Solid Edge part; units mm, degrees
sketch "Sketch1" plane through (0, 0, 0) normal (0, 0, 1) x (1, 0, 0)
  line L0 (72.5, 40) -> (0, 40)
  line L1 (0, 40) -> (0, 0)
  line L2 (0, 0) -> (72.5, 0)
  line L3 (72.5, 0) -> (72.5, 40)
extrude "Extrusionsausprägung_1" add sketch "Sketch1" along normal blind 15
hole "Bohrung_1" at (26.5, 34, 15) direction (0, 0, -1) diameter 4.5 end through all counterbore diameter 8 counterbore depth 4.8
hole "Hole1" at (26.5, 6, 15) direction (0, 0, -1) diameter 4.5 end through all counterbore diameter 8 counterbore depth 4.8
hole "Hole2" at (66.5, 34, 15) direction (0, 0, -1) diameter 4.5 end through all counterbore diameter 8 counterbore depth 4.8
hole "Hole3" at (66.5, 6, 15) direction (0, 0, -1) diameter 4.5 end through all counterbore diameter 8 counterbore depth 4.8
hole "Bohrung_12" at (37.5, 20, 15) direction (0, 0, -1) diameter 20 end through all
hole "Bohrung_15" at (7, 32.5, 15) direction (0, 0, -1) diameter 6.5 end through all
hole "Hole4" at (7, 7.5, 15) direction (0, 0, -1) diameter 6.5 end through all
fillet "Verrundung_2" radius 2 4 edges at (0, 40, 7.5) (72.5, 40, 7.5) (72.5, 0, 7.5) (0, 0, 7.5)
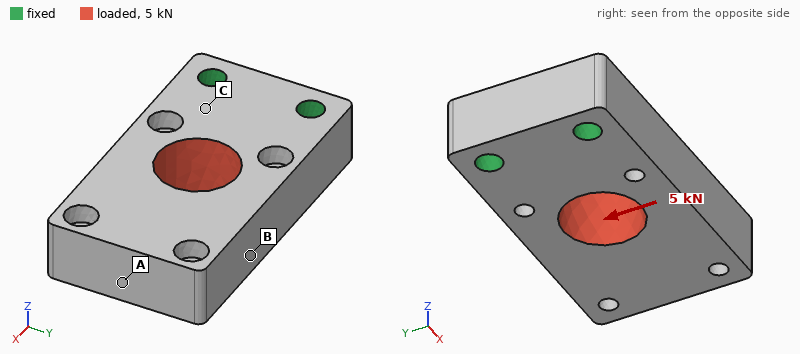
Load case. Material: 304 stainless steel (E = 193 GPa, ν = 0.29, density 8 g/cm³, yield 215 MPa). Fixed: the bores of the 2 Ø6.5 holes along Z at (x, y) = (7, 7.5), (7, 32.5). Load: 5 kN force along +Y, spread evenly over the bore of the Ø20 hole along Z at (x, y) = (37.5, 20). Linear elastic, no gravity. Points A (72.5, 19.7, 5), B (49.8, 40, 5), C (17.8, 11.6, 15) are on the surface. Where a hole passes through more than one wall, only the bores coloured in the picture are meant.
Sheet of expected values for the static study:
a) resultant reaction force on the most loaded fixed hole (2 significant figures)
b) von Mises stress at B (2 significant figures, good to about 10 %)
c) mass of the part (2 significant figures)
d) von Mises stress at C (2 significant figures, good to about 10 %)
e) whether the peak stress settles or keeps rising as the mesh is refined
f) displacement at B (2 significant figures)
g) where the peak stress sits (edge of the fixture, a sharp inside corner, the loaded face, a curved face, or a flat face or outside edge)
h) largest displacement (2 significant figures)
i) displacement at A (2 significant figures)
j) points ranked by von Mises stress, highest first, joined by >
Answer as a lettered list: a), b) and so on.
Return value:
a) 5.7 kN
b) 12 MPa
c) 290 g
d) 21 MPa
e) keeps rising
f) 16 µm
g) edge of the fixture
h) 20 µm
i) 20 µm
j) C > B > A
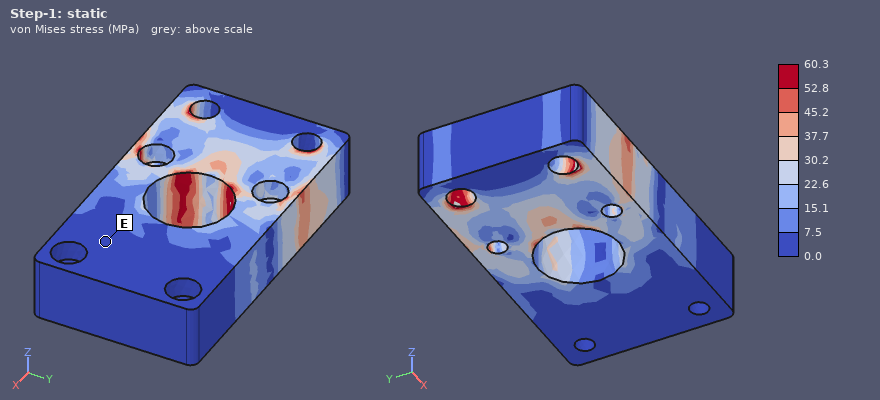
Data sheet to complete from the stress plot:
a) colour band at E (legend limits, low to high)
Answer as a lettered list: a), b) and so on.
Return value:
a) 0.0 to 7.5 MPa
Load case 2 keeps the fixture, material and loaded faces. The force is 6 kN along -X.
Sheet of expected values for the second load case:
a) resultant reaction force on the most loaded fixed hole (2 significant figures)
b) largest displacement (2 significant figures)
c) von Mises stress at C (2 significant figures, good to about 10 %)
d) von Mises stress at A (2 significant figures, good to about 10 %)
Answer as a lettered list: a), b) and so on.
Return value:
a) 3.0 kN
b) 4.4 µm
c) 13 MPa
d) 3.7 MPa
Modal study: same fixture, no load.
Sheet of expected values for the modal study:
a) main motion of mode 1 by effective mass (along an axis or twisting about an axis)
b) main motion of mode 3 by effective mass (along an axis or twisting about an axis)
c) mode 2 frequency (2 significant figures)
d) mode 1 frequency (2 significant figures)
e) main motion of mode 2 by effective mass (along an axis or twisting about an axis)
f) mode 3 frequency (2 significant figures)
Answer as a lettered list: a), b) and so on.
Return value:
a) along Z
b) twisting about X
c) 5000 Hz
d) 2300 Hz
e) along Y
f) 6900 Hz
